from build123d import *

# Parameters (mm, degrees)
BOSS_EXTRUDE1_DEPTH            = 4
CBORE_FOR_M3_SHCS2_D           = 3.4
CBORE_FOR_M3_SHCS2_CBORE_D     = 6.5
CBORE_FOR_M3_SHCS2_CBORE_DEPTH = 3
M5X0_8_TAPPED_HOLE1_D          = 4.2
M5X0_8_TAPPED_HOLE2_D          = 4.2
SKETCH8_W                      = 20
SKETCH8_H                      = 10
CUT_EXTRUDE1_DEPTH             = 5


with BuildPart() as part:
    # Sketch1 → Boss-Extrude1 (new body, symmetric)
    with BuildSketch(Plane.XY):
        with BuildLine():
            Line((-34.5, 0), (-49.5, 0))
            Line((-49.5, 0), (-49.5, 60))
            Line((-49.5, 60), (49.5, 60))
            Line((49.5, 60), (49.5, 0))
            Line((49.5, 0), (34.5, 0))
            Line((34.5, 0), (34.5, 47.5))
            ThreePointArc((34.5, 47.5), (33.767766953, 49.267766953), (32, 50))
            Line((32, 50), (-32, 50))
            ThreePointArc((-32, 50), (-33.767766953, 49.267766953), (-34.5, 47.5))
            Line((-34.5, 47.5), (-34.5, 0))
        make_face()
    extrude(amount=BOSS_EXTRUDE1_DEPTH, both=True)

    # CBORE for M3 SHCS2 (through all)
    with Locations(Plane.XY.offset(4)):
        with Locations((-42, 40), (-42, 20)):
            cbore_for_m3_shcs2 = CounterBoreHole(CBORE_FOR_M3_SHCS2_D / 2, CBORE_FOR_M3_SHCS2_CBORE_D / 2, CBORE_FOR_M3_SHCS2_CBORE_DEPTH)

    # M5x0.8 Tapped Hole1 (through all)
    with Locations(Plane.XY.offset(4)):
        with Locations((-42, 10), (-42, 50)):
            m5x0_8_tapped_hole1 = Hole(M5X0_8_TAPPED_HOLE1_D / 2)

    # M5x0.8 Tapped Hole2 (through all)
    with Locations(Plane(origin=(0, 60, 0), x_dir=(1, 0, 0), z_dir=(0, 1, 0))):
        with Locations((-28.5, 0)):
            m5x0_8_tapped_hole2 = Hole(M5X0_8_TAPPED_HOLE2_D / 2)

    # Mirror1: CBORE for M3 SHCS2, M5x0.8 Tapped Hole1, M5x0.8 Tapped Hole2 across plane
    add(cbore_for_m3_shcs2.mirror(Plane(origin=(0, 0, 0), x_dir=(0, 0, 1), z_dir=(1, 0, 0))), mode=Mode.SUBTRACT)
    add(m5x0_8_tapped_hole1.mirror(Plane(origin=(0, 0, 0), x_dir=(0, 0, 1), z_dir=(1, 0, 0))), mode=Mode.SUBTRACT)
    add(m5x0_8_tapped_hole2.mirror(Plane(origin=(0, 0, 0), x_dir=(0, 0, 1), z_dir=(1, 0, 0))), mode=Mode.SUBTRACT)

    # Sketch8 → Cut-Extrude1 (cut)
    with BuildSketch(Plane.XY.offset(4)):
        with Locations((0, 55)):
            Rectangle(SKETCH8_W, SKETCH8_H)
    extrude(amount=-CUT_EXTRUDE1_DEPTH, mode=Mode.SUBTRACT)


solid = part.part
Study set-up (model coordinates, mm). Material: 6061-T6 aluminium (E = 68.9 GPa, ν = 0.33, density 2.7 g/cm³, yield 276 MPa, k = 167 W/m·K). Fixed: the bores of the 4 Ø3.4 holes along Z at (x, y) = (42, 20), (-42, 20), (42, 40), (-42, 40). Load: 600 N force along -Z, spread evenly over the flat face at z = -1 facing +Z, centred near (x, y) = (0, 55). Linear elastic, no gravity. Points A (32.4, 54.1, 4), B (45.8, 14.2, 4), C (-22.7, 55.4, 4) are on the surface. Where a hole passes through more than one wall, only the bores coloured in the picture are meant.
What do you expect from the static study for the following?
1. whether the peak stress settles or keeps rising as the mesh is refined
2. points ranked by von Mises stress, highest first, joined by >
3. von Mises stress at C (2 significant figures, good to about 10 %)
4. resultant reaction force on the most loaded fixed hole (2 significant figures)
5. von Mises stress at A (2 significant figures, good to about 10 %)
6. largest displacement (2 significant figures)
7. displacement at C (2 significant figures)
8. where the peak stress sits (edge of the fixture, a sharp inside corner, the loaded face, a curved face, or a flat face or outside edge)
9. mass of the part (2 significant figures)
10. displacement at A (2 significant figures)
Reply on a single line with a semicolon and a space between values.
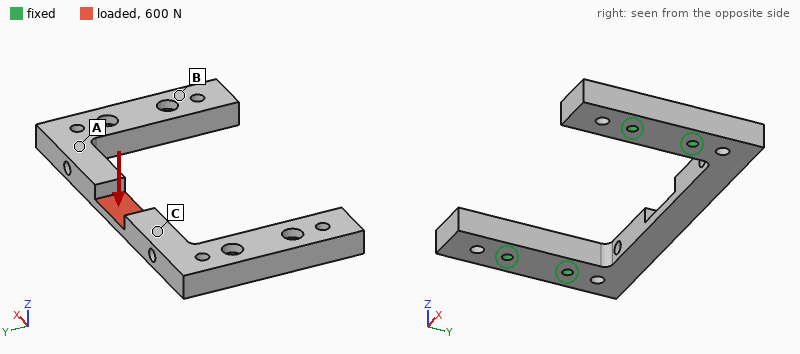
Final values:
keeps rising; A > C > B; 31 MPa; 750 N; 66 MPa; 0.27 mm; 0.13 mm; edge of the fixture; 48 g; 0.066 mm
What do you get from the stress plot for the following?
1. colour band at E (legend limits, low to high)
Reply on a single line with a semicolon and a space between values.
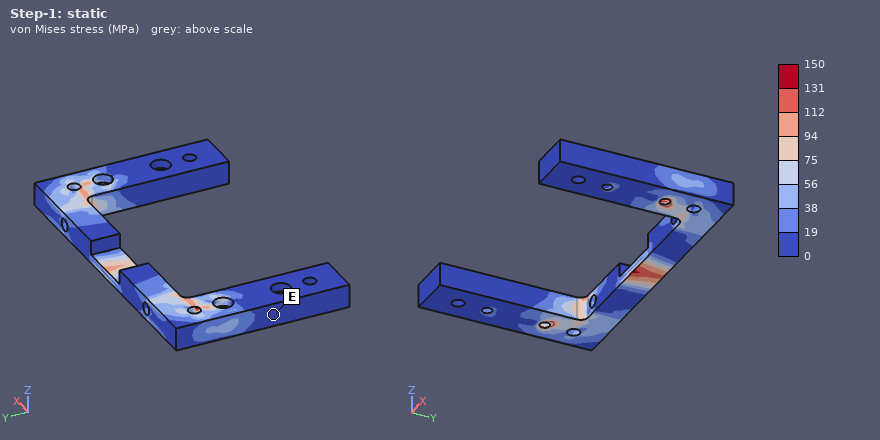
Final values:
0 to 19 MPa
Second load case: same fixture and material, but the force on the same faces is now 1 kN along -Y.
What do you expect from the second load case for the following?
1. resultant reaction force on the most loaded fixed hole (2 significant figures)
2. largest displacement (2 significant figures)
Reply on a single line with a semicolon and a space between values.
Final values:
530 N; 0.12 mm
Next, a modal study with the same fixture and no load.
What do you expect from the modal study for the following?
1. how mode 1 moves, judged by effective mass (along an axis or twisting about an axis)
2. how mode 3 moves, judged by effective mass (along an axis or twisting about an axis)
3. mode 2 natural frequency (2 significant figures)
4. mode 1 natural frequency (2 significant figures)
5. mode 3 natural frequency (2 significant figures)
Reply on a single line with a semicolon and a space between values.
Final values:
along Z; along Y; 6800 Hz; 3400 Hz; 7100 Hz
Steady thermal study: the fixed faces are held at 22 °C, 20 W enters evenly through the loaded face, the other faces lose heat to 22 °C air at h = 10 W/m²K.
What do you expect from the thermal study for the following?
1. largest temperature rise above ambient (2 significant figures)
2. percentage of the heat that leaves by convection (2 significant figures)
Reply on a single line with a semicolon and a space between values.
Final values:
45 K; 3.6 %
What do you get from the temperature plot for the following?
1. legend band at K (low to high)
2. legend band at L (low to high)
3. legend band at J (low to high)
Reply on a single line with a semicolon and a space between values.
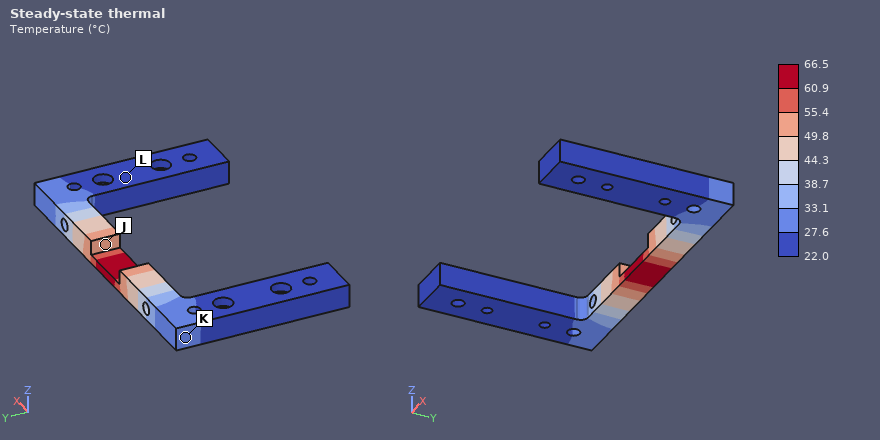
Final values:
27.6 to 33.1 °C; 22.0 to 27.6 °C; 49.8 to 55.4 °C
